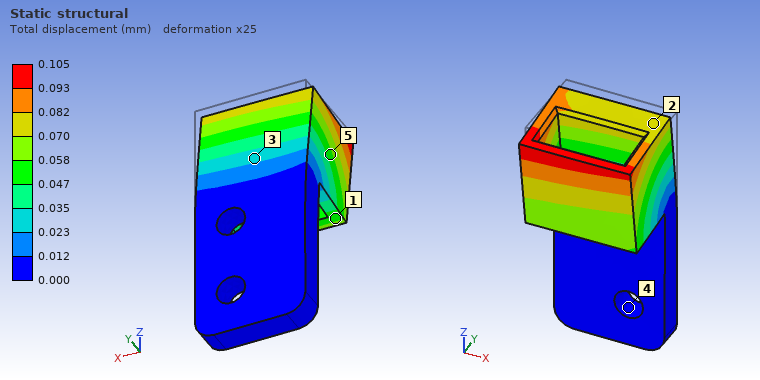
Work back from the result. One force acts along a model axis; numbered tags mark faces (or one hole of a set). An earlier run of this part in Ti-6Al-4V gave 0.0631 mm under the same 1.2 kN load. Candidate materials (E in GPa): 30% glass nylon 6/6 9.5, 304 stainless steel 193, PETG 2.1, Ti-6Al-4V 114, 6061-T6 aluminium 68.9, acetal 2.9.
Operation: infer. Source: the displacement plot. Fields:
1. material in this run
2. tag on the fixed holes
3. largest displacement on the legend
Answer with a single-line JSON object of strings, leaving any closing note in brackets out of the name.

{"material in this run": "6061-T6 aluminium", "tag on the fixed holes": "4", "largest displacement on the legend": "0.105 mm"}
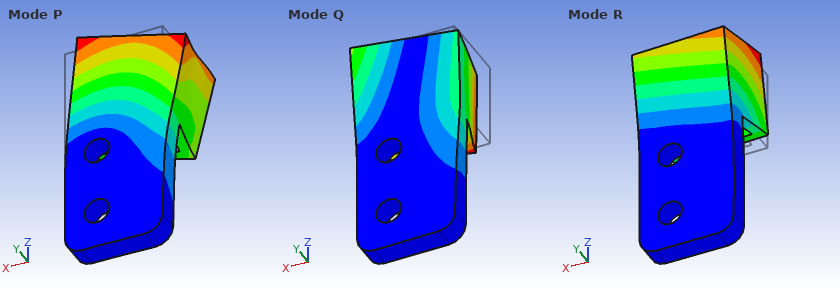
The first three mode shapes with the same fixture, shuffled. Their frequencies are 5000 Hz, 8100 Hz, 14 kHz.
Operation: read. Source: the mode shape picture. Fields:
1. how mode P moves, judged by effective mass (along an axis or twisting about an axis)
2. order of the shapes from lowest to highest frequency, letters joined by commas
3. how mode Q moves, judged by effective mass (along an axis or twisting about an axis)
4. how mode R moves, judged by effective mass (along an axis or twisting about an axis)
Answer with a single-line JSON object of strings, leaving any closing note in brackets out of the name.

{"how mode P moves, judged by effective mass": "along X", "order of the shapes from lowest to highest frequency, letters joined by commas": "R, Q, P", "how mode Q moves, judged by effective mass": "along X", "how mode R moves, judged by effective mass": "along Y"}
